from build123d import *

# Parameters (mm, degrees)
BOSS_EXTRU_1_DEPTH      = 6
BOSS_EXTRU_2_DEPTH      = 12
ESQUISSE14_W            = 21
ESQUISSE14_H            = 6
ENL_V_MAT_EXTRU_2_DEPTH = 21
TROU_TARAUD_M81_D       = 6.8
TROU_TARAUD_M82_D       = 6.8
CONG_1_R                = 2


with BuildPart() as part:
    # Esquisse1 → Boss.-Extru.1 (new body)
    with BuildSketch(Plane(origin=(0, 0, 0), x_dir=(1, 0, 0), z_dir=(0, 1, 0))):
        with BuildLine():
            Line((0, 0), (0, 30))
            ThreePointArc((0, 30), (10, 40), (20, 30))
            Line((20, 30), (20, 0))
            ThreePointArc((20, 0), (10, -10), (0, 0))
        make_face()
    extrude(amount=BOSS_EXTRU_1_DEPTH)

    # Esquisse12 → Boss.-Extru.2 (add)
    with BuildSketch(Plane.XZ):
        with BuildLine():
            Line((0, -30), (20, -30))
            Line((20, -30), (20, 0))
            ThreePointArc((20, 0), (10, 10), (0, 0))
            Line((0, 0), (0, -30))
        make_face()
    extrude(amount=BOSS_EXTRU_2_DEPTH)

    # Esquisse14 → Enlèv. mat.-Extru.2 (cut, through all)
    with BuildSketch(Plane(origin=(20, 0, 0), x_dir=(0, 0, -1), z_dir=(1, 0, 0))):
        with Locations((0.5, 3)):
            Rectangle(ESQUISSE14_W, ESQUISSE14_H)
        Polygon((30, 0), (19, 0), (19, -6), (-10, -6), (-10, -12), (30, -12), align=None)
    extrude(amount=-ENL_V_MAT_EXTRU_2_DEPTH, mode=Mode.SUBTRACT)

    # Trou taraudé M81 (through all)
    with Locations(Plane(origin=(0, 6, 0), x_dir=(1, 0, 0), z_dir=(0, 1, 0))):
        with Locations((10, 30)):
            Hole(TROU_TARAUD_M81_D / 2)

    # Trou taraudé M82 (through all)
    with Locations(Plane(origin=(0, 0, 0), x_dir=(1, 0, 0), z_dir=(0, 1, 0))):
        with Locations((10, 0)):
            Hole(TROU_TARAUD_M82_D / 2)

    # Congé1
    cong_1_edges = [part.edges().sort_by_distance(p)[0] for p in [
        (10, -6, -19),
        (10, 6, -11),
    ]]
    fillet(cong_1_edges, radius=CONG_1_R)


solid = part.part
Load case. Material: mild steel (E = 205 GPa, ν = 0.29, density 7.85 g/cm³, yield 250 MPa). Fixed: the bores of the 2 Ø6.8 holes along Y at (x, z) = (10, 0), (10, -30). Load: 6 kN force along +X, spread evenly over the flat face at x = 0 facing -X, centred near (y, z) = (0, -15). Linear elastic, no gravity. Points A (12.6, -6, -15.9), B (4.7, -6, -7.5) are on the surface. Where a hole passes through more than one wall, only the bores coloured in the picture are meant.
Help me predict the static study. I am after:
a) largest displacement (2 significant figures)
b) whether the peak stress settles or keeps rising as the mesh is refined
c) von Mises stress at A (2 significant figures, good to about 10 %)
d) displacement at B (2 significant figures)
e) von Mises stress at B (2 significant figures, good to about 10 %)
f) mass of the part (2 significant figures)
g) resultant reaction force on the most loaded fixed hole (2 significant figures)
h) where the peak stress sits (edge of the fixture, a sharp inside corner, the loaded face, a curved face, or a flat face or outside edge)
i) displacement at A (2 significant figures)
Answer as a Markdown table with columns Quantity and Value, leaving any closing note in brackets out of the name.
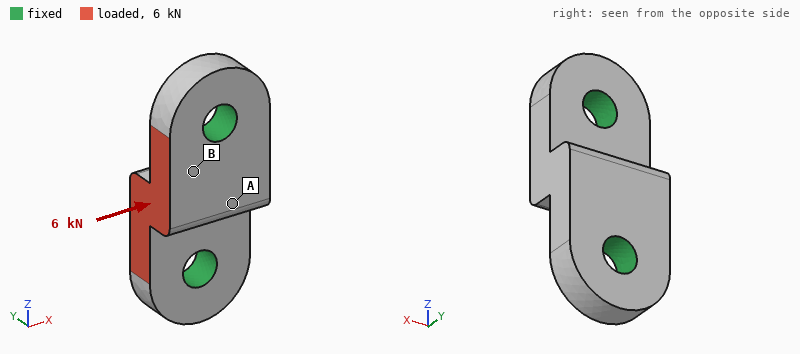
| Quantity | Value |
|---|---|
| largest displacement | 5.4 µm |
| whether the peak stress settles or keeps rising as the mesh is refined | keeps rising |
| von Mises stress at A | 14 MPa |
| displacement at B | 2.9 µm |
| von Mises stress at B | 36 MPa |
| mass of the part | 47 g |
| resultant reaction force on the most loaded fixed hole | 3.0 kN |
| where the peak stress sits | edge of the fixture |
| displacement at A | 3.9 µm |
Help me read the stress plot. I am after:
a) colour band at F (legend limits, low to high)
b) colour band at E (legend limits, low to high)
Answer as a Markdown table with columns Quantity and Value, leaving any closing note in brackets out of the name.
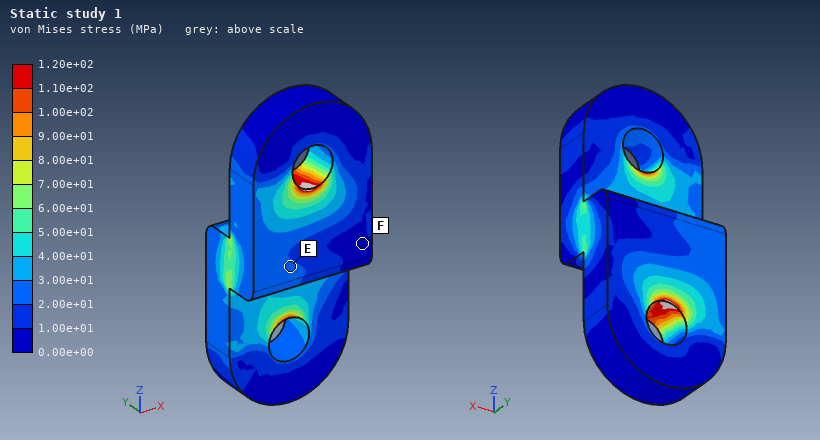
| Quantity | Value |
|---|---|
| colour band at F | 0.00e+00 to 1.00e+01 MPa |
| colour band at E | 2.00e+01 to 3.00e+01 MPa |
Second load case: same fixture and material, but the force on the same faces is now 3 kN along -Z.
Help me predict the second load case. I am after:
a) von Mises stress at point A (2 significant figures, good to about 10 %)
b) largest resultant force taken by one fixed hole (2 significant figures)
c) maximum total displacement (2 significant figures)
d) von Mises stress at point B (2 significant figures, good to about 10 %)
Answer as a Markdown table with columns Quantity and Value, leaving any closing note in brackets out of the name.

| Quantity | Value |
|---|---|
| von Mises stress at point A | 6.7 MPa |
| largest resultant force taken by one fixed hole | 1.7 kN |
| maximum total displacement | 4.3 µm |
| von Mises stress at point B | 17 MPa |
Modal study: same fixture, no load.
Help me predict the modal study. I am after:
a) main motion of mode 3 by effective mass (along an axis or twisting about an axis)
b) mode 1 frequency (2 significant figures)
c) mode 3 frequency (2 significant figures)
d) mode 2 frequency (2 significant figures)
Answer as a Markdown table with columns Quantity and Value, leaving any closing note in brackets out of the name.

| Quantity | Value |
|---|---|
| main motion of mode 3 by effective mass | along X |
| mode 1 frequency | 26 kHz |
| mode 3 frequency | 34 kHz |
| mode 2 frequency | 27 kHz |
